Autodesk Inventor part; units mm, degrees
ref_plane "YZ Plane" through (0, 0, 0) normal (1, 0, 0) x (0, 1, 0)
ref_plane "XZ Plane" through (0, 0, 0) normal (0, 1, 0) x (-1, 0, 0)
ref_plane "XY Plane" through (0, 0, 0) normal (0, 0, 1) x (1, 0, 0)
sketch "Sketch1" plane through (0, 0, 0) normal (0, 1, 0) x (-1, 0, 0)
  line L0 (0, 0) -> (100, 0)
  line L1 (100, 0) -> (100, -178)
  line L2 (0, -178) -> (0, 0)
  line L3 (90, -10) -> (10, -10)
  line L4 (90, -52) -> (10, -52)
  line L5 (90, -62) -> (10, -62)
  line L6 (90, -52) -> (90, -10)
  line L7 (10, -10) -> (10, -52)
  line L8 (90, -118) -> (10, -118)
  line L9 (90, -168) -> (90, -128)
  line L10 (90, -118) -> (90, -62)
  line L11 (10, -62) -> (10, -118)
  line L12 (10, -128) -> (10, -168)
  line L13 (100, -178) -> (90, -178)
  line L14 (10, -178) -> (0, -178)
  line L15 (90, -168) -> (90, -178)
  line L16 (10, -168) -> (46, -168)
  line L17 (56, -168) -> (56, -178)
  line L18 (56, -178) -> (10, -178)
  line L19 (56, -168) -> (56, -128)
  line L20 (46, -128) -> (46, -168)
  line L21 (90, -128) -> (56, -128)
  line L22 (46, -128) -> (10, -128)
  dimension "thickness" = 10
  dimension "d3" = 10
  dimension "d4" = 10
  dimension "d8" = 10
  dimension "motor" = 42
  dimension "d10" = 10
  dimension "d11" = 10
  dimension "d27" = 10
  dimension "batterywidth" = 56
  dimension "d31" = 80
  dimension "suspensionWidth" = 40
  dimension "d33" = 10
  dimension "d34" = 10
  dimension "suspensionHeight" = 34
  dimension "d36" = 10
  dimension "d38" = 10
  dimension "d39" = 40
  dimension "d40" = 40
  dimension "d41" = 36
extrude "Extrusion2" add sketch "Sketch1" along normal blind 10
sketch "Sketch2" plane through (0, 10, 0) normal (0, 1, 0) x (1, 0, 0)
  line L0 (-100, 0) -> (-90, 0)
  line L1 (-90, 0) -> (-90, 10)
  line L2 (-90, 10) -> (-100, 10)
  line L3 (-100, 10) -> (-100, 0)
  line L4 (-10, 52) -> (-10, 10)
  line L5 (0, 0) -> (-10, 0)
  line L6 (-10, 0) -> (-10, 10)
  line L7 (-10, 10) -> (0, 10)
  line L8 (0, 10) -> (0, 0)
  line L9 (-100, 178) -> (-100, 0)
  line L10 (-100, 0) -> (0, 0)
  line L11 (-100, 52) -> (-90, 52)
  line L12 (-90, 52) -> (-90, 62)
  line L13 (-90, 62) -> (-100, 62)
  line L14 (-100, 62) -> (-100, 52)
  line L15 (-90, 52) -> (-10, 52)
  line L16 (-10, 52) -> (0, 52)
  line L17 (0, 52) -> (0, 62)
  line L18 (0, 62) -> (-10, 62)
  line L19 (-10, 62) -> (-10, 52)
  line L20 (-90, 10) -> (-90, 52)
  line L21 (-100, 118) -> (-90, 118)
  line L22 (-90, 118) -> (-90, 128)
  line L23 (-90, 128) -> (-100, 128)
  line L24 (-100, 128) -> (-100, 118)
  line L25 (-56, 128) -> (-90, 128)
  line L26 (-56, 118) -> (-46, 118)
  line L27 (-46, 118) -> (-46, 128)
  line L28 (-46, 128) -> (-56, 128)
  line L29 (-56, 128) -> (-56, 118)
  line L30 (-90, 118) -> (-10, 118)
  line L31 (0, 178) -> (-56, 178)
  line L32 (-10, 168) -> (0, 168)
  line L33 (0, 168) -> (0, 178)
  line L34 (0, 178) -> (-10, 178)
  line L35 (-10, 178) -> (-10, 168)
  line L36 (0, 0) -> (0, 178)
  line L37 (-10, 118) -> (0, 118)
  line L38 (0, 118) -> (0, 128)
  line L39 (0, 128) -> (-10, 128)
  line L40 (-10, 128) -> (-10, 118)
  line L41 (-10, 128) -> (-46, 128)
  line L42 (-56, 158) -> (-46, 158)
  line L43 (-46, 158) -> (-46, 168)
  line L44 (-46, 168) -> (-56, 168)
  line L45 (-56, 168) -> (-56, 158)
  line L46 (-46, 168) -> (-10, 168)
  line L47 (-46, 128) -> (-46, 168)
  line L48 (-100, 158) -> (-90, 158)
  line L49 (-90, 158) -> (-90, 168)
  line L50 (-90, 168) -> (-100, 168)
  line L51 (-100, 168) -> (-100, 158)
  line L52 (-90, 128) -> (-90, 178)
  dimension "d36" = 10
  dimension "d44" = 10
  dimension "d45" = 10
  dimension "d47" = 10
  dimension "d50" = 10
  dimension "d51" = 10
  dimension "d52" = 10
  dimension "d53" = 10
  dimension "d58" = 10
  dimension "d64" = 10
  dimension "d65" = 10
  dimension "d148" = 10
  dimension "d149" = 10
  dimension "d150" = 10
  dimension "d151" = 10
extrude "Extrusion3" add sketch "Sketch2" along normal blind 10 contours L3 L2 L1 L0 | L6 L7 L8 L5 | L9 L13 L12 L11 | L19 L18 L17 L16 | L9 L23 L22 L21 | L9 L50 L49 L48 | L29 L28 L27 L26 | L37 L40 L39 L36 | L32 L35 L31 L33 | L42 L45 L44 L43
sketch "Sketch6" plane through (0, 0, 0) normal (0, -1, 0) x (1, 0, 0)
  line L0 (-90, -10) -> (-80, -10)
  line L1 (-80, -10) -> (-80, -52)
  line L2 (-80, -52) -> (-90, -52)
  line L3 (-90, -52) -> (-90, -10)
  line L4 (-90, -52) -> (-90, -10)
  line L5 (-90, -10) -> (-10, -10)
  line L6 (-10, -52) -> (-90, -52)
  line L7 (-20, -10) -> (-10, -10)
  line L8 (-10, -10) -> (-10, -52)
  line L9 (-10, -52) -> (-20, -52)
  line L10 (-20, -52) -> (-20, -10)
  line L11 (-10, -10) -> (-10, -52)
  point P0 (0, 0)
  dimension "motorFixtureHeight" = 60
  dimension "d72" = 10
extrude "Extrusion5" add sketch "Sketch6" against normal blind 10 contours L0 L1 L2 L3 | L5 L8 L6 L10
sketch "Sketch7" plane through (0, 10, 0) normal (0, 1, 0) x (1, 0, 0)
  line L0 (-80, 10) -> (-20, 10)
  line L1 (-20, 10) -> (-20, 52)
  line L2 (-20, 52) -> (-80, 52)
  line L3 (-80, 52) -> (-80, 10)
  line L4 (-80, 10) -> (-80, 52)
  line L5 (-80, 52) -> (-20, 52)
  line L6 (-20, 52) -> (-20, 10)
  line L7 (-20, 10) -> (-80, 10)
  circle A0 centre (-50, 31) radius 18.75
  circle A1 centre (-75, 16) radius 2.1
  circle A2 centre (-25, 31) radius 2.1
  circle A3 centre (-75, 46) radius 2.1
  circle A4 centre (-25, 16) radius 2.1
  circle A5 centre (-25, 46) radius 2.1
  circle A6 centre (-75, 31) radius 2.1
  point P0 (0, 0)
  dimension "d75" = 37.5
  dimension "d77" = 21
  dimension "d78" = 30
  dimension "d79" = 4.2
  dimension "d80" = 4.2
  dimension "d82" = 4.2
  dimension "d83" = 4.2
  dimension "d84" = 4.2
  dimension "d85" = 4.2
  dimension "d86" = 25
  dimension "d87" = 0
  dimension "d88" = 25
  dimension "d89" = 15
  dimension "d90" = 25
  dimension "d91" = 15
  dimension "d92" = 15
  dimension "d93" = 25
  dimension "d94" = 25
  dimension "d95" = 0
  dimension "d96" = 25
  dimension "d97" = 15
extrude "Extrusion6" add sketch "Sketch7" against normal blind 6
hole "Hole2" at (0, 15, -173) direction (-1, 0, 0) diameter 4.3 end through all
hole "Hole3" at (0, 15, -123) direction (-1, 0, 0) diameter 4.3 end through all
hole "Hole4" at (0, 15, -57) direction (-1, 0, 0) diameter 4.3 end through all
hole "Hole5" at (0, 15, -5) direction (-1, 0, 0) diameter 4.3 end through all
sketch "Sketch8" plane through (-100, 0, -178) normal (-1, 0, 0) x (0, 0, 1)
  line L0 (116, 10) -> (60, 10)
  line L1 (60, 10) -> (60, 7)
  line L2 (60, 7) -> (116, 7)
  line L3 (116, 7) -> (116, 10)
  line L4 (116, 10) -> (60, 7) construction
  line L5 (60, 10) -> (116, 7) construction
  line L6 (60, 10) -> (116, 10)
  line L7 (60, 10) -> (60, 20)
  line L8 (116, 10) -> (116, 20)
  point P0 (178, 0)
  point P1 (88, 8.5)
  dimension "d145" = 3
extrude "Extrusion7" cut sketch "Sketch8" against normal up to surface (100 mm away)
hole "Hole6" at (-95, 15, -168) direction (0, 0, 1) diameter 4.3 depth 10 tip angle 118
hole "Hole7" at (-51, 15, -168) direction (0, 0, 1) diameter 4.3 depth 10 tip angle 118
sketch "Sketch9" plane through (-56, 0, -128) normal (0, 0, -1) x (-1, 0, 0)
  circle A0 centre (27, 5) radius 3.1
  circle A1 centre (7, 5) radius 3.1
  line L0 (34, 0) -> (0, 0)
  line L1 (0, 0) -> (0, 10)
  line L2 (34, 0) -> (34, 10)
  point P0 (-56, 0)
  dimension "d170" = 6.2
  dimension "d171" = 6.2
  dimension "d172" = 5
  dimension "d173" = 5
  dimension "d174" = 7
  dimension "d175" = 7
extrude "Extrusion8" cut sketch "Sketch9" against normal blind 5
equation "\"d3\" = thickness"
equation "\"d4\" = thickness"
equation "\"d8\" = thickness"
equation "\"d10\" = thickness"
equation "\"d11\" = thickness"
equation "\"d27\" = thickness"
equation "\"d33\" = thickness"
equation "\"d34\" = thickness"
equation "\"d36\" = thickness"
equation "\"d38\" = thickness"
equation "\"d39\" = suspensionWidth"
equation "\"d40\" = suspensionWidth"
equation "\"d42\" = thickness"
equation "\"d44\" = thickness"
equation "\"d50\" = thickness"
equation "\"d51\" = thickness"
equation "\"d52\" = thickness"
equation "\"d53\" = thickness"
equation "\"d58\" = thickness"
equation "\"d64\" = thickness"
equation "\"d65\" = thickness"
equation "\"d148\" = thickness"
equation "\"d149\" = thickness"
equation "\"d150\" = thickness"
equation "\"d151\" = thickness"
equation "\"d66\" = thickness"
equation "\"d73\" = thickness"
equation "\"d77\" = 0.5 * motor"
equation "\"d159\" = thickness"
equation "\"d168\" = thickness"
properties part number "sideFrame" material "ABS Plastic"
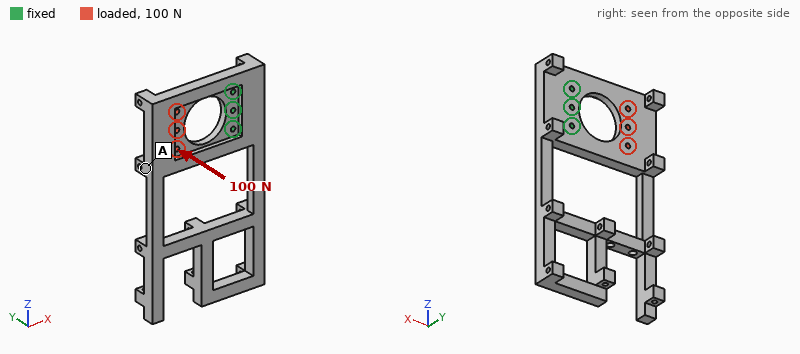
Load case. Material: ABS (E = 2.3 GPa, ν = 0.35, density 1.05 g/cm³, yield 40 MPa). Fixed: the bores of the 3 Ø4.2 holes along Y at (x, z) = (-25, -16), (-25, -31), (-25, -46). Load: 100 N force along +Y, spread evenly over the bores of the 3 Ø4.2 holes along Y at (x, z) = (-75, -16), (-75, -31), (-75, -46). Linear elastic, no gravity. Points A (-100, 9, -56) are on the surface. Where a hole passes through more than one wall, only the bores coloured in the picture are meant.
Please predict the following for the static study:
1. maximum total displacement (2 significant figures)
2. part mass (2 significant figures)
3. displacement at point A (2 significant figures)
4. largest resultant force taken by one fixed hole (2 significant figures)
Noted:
2.2 mm
94 g
2.1 mm
80 N
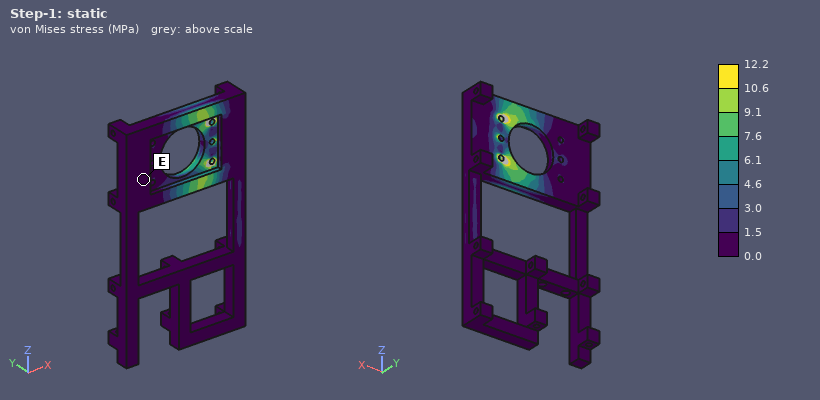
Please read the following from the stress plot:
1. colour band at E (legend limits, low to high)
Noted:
0.0 to 1.5 MPa
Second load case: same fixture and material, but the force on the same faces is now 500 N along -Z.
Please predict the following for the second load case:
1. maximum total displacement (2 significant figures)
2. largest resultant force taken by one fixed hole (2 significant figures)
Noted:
1.5 mm
740 N
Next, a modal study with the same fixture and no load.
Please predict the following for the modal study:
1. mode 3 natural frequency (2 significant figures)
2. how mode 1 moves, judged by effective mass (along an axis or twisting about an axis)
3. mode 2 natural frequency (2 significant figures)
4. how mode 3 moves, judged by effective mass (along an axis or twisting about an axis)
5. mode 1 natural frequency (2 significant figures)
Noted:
200 Hz
along Y
130 Hz
along X
55 Hz
